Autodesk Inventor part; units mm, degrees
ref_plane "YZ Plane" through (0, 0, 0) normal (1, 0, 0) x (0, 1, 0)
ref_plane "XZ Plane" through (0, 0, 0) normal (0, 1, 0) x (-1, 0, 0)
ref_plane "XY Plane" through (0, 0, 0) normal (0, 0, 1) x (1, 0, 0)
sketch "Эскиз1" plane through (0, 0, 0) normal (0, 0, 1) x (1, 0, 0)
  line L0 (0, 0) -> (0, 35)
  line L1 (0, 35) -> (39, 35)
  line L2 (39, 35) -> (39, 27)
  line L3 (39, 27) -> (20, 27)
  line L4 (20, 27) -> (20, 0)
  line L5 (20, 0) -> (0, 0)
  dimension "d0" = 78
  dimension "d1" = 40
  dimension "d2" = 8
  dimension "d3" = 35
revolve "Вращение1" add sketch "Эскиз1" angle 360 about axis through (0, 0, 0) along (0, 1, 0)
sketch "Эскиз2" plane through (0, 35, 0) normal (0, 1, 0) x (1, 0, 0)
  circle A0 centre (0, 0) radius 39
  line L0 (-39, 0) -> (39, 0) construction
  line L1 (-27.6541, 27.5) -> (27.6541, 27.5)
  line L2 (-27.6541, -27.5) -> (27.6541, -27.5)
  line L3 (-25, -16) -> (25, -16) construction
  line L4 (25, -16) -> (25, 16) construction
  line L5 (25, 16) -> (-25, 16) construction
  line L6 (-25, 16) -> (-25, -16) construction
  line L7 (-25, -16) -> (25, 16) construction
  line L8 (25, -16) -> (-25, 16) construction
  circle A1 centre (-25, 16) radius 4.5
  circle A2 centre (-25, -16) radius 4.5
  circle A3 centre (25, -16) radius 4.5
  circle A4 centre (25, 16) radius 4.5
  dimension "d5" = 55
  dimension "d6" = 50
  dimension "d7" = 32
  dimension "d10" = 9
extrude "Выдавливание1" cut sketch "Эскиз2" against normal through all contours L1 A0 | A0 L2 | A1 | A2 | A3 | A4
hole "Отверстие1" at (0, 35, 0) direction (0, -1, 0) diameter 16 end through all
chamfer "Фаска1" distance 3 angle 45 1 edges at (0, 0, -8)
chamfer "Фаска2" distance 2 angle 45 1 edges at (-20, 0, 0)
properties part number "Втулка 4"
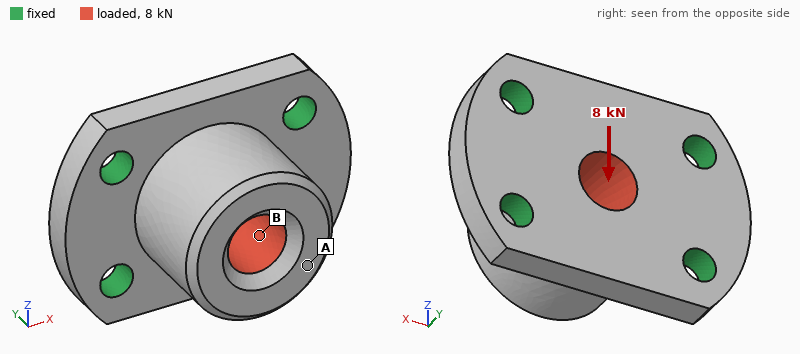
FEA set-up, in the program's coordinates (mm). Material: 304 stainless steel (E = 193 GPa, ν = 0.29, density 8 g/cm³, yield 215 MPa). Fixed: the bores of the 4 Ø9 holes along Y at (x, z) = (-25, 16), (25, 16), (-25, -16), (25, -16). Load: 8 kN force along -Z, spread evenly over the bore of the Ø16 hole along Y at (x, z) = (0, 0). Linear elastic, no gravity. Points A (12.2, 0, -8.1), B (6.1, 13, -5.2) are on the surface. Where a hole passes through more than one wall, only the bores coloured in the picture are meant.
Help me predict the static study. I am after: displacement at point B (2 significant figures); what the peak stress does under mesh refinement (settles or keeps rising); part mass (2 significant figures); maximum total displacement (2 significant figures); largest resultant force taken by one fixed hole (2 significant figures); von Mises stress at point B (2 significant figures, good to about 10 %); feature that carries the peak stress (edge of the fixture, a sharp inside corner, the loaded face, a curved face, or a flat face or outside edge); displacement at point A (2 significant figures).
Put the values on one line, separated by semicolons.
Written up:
5.9 µm; keeps rising; 440 g; 9.4 µm; 2.7 kN; 10 MPa; edge of the fixture; 8.6 µm
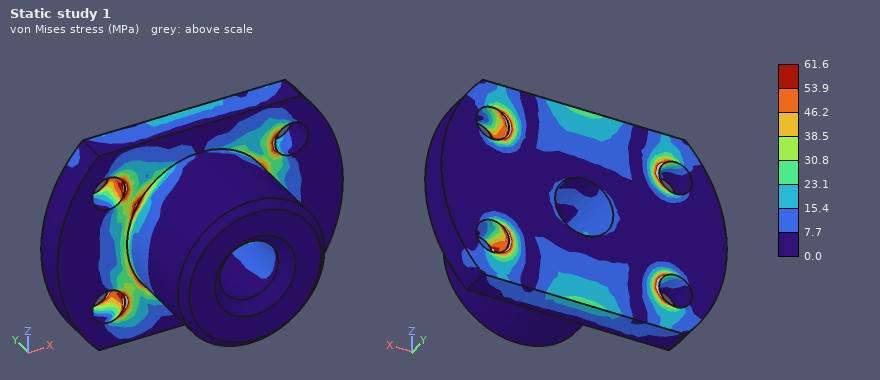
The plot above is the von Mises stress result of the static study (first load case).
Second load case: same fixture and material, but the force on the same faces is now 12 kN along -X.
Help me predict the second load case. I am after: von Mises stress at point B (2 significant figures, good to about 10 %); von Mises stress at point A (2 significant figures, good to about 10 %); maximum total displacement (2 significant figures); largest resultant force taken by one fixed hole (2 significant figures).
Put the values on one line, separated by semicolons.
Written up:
14 MPa; 5.7 MPa; 8.0 µm; 3.6 kN
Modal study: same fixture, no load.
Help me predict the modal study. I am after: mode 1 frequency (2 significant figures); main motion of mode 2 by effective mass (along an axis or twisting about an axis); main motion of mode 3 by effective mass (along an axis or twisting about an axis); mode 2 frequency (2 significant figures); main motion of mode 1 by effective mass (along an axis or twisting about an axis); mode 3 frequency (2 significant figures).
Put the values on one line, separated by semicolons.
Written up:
9000 Hz; along X; along Y; 12 kHz; along Z; 13 kHz
